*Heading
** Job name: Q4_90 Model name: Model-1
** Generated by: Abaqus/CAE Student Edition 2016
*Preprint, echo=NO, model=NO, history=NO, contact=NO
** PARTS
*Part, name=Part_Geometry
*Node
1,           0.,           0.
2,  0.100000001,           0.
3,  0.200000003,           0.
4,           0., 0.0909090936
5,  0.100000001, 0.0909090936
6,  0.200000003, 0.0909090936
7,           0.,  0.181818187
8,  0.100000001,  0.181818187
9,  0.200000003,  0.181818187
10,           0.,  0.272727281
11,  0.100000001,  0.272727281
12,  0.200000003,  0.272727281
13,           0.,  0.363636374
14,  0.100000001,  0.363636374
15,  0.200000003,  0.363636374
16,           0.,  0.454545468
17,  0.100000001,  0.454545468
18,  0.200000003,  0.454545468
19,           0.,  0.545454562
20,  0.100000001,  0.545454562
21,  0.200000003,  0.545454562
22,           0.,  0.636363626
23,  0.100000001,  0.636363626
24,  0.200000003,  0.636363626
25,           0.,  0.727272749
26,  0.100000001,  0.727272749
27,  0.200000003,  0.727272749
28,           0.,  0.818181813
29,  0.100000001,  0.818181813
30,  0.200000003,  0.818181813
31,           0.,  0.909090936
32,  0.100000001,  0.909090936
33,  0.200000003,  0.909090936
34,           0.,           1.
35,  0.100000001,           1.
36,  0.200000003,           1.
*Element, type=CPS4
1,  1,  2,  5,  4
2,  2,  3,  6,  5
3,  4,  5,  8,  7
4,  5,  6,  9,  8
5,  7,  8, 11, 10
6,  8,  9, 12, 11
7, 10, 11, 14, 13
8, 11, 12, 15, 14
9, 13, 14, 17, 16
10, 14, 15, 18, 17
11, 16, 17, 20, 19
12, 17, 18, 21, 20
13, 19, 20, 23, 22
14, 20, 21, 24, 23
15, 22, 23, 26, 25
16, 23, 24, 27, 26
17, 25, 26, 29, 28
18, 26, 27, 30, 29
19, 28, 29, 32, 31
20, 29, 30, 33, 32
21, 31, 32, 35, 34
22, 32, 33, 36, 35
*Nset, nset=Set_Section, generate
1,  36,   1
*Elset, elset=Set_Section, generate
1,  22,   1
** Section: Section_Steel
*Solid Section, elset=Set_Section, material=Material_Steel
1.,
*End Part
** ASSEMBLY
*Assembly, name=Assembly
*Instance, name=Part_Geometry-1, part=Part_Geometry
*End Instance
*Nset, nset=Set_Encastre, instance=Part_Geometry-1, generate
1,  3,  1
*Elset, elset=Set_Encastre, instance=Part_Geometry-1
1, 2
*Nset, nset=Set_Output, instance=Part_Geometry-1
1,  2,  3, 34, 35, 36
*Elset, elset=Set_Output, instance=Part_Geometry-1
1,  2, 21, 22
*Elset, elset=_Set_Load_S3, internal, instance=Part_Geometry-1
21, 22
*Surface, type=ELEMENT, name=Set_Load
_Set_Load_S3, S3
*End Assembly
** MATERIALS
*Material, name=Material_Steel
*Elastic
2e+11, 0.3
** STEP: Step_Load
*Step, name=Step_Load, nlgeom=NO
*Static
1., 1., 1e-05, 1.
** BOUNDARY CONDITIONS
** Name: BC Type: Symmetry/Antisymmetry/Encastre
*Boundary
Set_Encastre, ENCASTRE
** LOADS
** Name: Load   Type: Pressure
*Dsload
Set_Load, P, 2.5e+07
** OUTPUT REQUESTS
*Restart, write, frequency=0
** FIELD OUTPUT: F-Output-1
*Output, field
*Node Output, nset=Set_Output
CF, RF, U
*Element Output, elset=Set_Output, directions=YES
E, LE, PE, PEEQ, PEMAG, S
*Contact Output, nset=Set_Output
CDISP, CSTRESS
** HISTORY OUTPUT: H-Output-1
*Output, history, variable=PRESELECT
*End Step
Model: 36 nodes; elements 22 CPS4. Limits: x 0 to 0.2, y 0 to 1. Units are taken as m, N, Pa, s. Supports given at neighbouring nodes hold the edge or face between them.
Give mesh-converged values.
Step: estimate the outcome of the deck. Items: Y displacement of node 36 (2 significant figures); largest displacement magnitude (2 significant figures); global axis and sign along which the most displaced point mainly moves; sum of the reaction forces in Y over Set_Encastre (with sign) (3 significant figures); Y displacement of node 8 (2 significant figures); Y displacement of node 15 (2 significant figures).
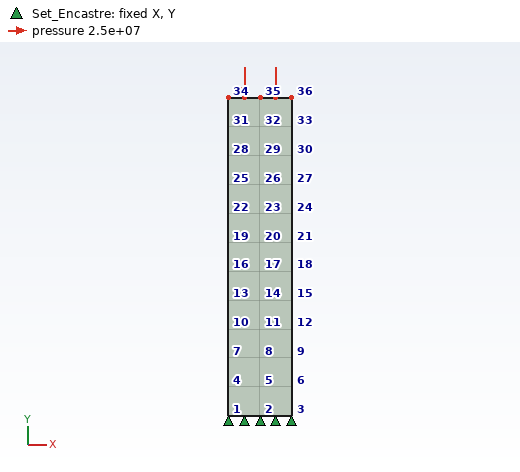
-1.2e-04 m
1.2e-04 m
-Y
5.00e+06 N
-2.2e-05 m
-4.5e-05 m
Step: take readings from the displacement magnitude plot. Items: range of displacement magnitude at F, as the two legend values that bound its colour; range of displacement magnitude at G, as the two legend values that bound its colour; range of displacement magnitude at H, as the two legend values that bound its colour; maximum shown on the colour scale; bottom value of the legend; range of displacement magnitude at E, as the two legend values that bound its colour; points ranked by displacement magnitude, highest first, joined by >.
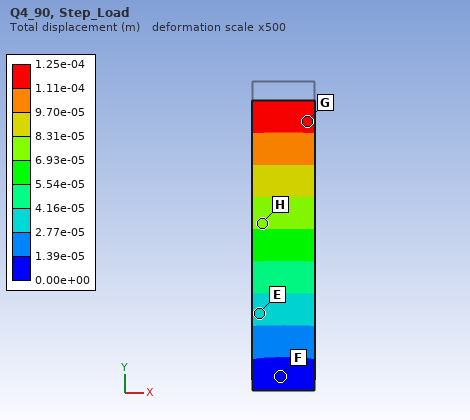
0.00e+00 to 1.39e-05 m
1.11e-04 to 1.25e-04 m
6.93e-05 to 8.31e-05 m
1.25e-04 m
0.00e+00 m
2.77e-05 to 4.16e-05 m
G > H > E > F
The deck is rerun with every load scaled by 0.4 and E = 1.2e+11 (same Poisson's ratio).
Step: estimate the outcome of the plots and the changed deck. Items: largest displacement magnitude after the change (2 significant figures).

8.3e-05 m
